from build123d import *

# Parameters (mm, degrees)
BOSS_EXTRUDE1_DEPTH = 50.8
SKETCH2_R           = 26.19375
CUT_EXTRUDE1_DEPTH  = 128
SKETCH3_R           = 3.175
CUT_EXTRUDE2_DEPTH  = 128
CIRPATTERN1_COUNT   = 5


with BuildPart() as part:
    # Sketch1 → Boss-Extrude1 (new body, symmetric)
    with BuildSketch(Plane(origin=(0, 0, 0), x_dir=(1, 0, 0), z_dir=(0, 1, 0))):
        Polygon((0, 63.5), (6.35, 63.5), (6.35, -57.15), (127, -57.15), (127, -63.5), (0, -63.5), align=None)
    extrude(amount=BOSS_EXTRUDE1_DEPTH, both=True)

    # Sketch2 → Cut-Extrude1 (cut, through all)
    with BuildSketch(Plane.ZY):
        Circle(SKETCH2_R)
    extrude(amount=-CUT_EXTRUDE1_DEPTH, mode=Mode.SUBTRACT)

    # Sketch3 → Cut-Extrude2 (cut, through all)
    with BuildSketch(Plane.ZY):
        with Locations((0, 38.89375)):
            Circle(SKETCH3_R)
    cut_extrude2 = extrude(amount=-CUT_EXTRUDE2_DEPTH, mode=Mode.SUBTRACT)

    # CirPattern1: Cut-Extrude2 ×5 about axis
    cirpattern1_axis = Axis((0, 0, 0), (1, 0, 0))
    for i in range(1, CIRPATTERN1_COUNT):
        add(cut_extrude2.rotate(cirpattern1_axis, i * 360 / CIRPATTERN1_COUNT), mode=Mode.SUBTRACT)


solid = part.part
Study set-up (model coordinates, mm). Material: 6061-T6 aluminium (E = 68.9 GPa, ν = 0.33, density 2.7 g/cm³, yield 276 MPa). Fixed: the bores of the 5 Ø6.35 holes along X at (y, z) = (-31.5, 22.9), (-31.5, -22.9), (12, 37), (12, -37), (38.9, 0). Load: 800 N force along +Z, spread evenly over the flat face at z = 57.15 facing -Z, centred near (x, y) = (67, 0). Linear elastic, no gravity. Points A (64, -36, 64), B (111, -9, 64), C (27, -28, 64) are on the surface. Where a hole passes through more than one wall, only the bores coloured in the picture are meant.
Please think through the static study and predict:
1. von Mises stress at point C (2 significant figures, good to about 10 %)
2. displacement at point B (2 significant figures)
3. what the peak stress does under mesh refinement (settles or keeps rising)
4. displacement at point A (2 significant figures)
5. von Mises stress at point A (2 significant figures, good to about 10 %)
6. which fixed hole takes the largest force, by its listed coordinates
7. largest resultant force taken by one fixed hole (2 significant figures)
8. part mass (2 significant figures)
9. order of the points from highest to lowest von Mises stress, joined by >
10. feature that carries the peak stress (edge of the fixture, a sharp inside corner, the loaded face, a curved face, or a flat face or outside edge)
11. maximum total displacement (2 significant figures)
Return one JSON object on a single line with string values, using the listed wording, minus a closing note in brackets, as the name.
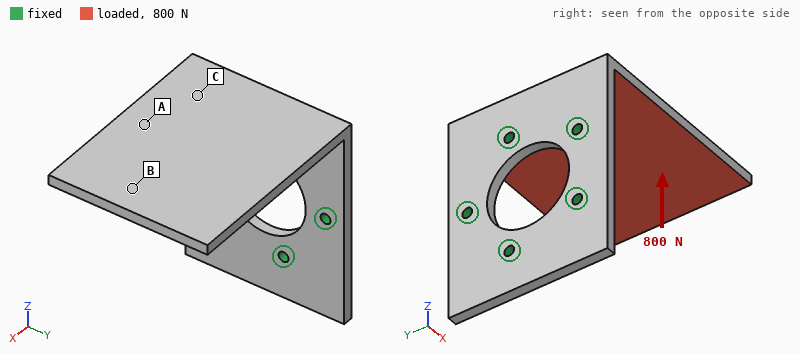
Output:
{"von Mises stress at point C": "42 MPa", "displacement at point B": "1.9 mm", "what the peak stress does under mesh refinement": "keeps rising", "displacement at point A": "0.96 mm", "von Mises stress at point A": "19 MPa", "which fixed hole takes the largest force, by its listed coordinates": "(12, 37)", "largest resultant force taken by one fixed hole": "800 N", "part mass": "390 g", "order of the points from highest to lowest von Mises stress, joined by >": "C > A > B", "feature that carries the peak stress": "edge of the fixture", "maximum total displacement": "2.3 mm"}
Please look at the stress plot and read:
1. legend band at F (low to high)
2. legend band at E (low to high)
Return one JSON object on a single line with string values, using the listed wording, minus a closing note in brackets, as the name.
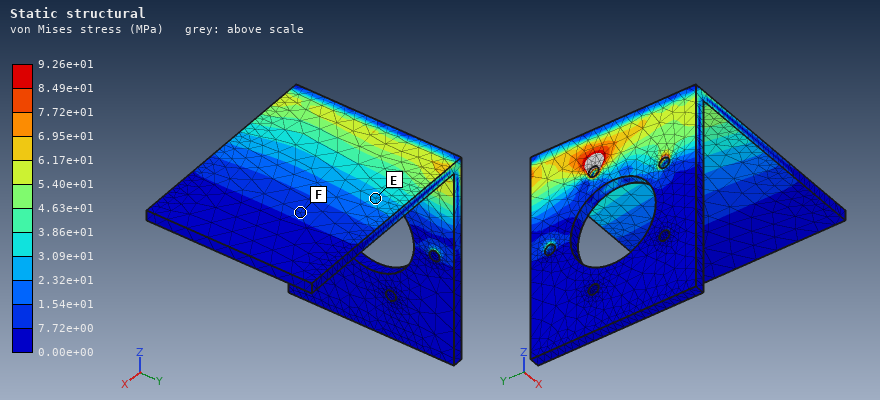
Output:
{"legend band at F": "7.72e+00 to 1.54e+01 MPa", "legend band at E": "2.32e+01 to 3.09e+01 MPa"}
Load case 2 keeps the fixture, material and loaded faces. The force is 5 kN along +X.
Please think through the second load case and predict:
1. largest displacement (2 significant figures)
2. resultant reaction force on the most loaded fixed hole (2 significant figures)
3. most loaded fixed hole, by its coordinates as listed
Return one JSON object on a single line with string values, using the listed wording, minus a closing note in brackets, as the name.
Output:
{"largest displacement": "0.98 mm", "resultant reaction force on the most loaded fixed hole": "4.5 kN", "most loaded fixed hole, by its coordinates as listed": "(12, 37)"}
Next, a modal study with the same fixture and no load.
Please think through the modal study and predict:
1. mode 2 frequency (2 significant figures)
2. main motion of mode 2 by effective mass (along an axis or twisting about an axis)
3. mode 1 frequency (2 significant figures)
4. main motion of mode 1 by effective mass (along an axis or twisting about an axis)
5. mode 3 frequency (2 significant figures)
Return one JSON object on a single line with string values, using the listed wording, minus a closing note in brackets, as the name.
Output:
{"mode 2 frequency": "570 Hz", "main motion of mode 2 by effective mass": "along Y", "mode 1 frequency": "250 Hz", "main motion of mode 1 by effective mass": "along Z", "mode 3 frequency": "940 Hz"}
